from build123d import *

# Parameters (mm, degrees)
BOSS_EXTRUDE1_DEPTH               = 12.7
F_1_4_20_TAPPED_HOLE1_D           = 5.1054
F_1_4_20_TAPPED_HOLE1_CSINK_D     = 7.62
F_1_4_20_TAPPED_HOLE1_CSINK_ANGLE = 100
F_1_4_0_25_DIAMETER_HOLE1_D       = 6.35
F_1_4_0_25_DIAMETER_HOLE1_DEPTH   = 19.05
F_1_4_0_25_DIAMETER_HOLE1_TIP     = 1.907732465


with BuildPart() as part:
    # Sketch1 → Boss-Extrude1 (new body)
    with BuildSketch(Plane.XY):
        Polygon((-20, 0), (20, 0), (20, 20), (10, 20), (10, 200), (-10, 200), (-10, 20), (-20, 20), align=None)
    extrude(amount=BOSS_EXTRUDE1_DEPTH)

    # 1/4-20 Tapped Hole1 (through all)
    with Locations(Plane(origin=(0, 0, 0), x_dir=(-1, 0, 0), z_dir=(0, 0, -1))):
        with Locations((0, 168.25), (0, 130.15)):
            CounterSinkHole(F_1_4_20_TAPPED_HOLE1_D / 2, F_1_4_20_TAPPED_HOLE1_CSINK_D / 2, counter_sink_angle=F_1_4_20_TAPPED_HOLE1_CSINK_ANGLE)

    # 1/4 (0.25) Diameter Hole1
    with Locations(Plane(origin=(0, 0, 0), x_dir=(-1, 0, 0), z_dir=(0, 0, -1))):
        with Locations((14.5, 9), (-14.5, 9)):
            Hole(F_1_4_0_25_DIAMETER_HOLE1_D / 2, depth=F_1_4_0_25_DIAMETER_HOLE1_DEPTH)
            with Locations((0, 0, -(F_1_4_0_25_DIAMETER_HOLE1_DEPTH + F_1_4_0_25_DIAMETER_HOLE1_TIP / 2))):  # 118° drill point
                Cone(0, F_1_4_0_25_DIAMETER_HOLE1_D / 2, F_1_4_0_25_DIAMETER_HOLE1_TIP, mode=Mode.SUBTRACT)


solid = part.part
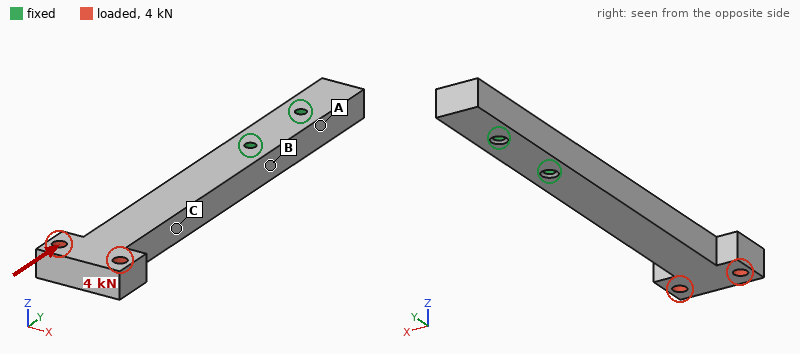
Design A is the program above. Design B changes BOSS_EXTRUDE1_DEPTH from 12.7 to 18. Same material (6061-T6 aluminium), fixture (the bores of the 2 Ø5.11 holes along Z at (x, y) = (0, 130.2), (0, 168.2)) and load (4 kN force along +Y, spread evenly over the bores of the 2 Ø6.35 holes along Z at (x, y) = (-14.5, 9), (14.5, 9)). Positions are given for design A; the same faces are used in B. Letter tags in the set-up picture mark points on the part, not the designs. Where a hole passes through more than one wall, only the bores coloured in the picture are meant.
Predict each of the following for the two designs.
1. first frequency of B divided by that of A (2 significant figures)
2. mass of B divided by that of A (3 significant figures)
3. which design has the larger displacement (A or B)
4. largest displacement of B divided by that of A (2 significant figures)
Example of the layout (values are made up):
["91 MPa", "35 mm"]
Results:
["1.4", "1.42", "A", "0.70"]
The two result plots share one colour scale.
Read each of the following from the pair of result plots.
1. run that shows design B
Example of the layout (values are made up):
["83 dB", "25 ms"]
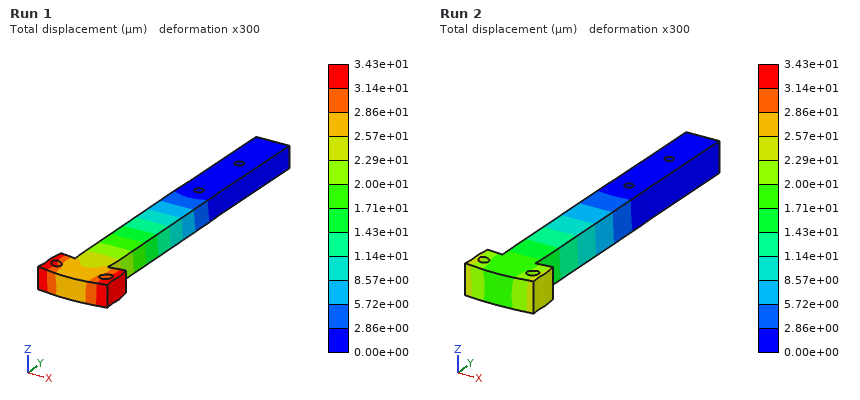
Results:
["Run 2"]
